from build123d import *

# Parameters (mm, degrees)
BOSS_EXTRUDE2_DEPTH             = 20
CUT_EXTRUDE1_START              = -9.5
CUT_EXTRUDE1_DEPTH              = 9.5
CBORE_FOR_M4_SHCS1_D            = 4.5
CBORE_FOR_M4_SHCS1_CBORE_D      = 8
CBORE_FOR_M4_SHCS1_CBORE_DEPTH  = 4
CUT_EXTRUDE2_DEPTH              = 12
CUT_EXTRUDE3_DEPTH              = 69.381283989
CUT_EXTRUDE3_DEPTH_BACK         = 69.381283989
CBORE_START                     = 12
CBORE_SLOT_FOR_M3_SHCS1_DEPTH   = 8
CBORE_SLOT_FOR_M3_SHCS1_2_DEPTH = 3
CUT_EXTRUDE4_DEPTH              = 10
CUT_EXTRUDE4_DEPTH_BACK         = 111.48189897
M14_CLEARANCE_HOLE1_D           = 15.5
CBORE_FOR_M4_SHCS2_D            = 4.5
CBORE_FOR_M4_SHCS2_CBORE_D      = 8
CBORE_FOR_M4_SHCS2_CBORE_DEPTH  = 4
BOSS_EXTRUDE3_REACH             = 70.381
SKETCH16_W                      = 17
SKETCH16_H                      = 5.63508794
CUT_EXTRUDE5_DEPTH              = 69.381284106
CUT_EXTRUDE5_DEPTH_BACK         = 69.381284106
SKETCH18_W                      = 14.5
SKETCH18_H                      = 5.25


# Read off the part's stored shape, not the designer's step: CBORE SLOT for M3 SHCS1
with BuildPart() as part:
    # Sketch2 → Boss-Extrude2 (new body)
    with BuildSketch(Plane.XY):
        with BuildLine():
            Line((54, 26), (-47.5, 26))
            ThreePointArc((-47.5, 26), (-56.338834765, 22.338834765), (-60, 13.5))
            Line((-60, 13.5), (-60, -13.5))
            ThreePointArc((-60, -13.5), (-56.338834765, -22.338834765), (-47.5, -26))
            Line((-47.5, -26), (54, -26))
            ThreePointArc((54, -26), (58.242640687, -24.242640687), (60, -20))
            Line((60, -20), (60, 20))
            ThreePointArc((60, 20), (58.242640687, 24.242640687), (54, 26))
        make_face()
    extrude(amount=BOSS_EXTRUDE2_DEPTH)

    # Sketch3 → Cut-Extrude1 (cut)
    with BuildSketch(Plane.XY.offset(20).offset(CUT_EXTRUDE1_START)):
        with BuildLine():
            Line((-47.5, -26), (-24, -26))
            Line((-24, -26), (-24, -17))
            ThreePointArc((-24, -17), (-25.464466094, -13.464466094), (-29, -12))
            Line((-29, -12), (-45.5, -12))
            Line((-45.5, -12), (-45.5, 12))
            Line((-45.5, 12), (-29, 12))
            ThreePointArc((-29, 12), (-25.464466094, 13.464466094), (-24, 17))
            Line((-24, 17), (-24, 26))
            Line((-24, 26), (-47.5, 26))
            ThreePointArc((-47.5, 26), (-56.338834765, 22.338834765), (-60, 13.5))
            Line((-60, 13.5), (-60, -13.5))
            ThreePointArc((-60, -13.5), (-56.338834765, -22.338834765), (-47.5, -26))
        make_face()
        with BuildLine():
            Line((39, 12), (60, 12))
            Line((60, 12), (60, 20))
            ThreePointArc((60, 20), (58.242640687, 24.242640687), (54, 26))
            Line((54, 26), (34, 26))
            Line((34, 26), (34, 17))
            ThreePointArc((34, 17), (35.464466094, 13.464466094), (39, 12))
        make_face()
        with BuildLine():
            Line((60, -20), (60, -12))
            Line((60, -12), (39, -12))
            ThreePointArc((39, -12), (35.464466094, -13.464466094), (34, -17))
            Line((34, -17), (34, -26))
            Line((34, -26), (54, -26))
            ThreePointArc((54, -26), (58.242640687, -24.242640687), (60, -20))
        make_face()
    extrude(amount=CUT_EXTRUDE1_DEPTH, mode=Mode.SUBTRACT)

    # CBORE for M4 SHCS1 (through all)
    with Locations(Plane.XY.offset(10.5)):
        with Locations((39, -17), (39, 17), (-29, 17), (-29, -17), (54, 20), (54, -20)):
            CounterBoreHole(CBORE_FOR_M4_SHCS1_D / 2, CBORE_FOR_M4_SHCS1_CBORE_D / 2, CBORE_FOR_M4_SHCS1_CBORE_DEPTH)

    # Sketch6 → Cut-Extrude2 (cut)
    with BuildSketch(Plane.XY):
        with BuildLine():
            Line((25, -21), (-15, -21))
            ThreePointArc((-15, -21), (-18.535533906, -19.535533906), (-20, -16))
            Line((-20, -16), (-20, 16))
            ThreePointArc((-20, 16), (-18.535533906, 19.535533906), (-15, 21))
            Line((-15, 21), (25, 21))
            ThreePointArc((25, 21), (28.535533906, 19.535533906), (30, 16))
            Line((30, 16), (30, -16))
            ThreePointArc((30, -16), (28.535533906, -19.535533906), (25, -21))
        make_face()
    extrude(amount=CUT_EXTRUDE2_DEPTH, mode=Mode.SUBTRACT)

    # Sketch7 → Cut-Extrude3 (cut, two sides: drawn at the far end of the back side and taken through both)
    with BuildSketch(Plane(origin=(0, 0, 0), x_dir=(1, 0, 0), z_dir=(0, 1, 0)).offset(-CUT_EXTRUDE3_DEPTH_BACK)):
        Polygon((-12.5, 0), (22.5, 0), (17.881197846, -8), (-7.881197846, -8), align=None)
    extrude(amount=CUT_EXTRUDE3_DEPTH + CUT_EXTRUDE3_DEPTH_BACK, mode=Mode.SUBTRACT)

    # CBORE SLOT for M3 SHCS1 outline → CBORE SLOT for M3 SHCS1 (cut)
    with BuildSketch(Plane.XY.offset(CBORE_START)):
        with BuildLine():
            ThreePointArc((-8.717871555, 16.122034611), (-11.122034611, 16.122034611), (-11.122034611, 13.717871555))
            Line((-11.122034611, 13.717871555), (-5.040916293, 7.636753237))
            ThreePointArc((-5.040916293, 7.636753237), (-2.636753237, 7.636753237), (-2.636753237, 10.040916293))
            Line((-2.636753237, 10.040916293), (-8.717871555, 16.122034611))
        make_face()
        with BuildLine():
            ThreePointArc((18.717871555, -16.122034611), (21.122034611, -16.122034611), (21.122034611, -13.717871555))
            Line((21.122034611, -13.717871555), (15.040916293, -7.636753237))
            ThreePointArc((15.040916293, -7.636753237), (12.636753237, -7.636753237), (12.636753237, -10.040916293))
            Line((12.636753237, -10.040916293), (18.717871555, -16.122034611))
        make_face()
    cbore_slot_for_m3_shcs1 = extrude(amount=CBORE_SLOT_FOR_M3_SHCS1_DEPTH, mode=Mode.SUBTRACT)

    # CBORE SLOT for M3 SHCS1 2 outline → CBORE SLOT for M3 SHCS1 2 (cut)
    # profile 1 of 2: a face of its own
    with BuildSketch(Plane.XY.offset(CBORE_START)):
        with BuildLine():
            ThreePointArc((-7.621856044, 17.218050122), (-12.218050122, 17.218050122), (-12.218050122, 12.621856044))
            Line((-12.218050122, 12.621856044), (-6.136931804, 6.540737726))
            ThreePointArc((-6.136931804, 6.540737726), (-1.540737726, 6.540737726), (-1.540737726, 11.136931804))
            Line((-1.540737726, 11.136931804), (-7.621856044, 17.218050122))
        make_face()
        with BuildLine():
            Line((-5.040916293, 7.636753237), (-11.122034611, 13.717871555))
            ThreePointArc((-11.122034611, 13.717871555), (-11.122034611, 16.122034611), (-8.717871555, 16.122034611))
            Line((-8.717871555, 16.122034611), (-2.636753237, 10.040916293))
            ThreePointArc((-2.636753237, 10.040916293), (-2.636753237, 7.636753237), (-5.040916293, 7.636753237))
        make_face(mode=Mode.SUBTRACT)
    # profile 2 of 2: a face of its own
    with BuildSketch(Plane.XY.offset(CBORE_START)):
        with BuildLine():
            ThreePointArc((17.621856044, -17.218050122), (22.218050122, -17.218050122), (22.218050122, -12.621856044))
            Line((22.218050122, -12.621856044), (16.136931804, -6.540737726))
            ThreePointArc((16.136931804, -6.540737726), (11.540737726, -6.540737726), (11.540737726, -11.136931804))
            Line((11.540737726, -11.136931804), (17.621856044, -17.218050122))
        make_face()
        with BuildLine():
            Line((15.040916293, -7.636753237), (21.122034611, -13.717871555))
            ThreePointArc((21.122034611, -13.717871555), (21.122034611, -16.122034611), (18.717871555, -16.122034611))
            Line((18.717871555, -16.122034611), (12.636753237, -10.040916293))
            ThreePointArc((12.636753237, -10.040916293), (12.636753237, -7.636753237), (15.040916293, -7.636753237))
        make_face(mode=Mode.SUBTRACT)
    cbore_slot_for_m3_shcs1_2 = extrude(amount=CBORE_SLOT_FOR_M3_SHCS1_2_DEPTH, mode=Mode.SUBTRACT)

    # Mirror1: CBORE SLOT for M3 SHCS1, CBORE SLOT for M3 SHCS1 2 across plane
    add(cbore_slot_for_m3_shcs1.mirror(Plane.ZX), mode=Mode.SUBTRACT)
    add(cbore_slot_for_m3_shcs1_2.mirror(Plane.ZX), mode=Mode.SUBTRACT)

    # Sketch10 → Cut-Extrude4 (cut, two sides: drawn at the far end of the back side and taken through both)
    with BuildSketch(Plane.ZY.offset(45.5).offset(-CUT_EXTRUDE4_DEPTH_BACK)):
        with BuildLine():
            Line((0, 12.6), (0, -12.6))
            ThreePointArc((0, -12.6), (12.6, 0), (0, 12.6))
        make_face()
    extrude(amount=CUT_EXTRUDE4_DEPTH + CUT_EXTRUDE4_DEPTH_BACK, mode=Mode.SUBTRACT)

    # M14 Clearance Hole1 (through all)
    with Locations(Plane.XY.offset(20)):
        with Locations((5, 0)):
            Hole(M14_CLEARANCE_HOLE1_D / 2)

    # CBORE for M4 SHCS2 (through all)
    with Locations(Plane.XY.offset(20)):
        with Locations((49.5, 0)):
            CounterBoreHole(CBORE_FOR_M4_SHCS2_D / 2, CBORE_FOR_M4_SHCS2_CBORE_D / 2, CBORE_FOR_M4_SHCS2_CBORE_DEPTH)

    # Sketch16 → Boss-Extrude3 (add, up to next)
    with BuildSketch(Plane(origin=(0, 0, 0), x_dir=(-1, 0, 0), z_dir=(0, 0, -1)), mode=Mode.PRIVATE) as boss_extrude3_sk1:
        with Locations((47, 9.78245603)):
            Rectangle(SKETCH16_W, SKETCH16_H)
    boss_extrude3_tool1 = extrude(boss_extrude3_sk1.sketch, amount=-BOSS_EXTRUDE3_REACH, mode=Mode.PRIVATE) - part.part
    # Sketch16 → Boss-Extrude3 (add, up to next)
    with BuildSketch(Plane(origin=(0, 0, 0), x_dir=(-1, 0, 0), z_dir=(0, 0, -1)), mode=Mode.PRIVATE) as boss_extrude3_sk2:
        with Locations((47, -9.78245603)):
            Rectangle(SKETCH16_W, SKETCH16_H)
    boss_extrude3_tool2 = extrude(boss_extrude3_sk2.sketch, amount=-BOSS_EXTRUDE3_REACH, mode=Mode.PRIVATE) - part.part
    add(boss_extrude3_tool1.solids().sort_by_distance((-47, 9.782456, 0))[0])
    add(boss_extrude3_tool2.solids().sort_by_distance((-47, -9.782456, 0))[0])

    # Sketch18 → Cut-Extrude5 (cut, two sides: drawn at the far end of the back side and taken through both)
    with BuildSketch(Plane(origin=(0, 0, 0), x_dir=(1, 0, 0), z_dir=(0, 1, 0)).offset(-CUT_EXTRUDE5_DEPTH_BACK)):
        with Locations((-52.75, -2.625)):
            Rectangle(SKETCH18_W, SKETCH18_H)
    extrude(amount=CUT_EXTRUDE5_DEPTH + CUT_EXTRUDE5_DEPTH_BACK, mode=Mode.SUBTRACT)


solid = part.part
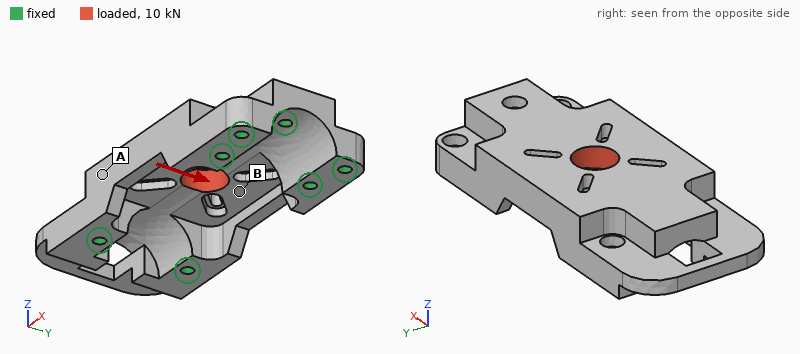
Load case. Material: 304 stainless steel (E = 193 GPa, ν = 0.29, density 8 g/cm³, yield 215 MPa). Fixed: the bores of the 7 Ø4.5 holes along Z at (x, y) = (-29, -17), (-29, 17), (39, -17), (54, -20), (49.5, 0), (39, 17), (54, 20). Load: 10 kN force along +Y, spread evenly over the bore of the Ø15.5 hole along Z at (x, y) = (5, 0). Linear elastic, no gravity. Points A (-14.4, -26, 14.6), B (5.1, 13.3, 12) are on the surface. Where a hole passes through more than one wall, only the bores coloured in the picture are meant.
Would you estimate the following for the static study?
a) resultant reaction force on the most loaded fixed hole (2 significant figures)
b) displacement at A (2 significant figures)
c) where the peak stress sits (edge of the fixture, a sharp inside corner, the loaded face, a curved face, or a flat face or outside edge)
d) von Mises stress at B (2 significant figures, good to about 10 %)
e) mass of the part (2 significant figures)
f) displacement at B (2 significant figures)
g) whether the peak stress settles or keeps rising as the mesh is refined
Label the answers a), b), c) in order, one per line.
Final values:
a) 2.8 kN
b) 8.3 µm
c) edge of the fixture
d) 16 MPa
e) 430 g
f) 13 µm
g) keeps rising
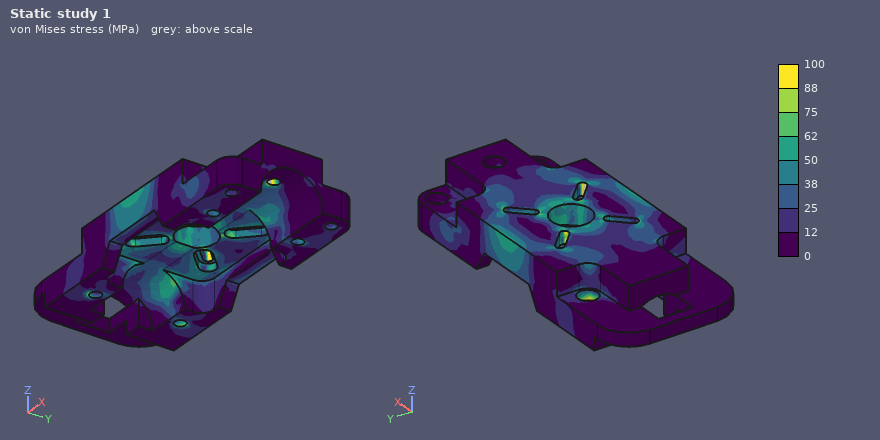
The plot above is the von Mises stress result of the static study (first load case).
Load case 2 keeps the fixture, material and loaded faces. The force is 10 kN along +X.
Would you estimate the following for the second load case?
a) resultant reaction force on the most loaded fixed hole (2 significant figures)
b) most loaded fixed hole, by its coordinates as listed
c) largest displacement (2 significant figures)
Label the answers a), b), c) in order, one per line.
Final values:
a) 2.5 kN
b) (49.5, 0)
c) 10 µm
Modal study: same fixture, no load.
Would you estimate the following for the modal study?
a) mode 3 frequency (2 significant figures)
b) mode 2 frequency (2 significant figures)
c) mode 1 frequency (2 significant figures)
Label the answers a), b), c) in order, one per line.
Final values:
a) 11 kHz
b) 11 kHz
c) 8300 Hz
